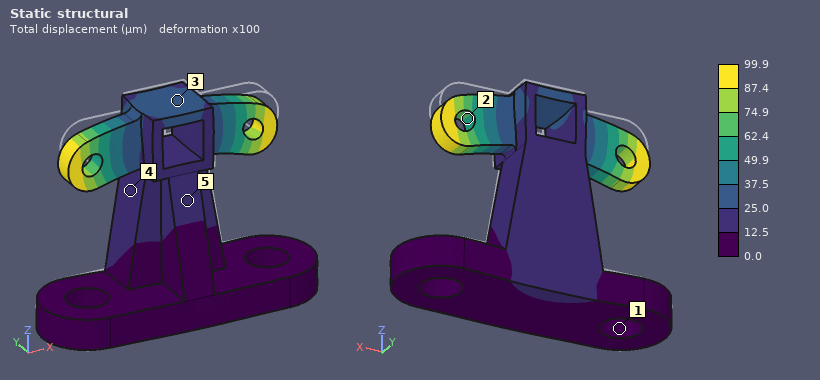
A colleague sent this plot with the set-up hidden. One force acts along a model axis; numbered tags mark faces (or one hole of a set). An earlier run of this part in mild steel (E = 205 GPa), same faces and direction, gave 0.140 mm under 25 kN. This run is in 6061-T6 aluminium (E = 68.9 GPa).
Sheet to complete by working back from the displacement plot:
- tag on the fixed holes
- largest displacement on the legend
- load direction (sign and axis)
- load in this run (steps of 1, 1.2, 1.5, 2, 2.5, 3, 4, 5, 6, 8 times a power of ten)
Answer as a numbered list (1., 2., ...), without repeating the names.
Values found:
1. 1
2. 99.9 µm
3. -Z
4. 6 kN
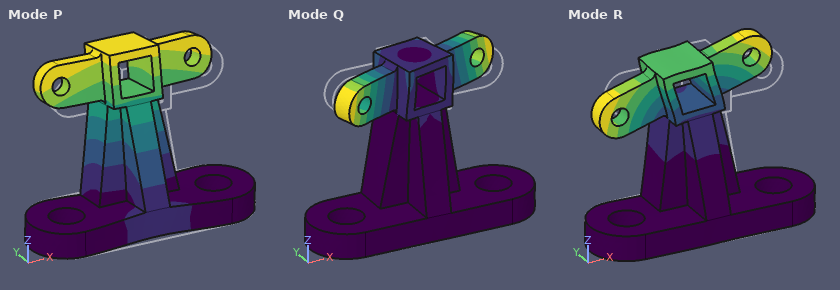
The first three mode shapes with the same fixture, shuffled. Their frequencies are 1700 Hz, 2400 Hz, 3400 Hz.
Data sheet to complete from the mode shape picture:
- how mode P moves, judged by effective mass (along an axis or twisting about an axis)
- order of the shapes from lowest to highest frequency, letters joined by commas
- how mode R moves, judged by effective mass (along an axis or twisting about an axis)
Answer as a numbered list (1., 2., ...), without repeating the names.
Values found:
1. along Y
2. P, R, Q
3. along X
